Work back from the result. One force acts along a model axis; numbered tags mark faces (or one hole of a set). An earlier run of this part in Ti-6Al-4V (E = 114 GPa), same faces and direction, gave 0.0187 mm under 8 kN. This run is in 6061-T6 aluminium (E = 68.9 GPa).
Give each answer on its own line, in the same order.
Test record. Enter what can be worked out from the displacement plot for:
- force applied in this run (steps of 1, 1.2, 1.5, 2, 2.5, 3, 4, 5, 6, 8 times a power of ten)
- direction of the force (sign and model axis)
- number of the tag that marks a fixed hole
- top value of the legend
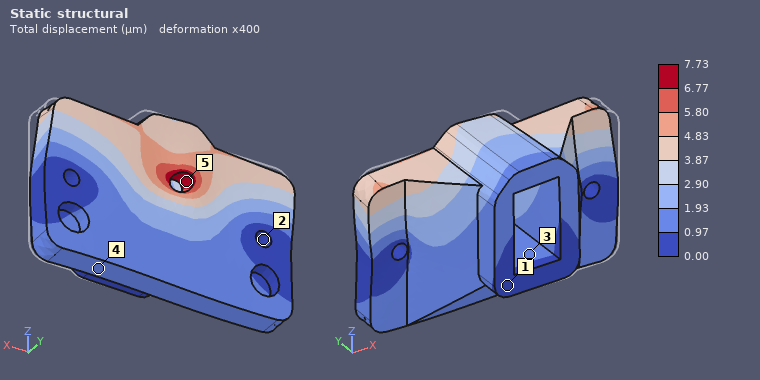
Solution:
2 kN
-X
2
7.73 µm
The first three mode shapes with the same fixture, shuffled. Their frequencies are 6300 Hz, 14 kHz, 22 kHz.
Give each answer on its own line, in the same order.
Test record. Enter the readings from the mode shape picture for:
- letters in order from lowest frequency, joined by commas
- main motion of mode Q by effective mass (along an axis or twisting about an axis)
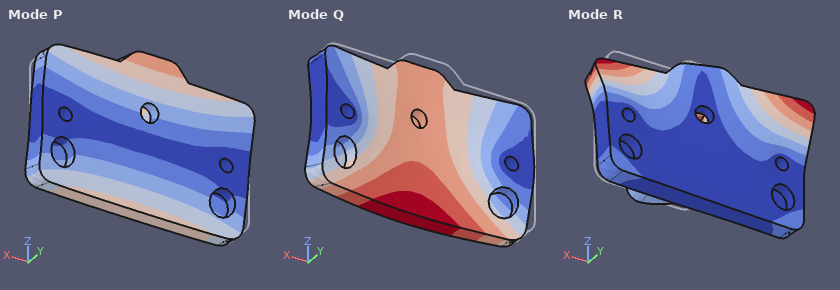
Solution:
P, Q, R
along Y
